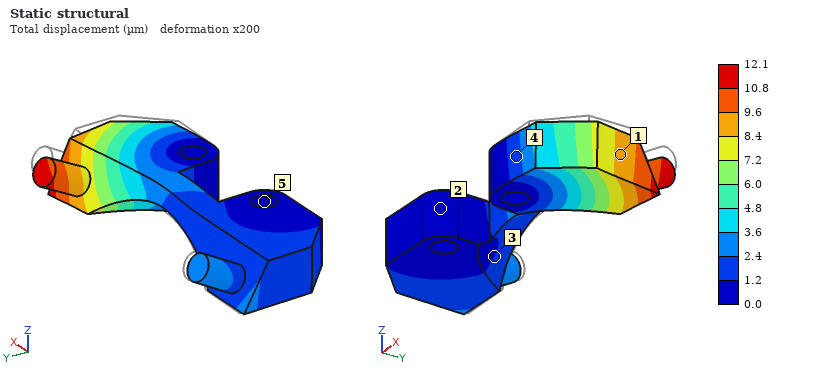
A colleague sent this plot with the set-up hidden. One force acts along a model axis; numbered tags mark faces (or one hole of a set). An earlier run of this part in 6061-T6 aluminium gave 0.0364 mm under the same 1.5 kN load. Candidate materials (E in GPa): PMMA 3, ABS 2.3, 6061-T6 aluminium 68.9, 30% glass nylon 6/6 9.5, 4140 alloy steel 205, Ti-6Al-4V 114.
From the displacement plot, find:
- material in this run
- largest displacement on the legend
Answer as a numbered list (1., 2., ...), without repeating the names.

1. 4140 alloy steel
2. 12.1 µm
